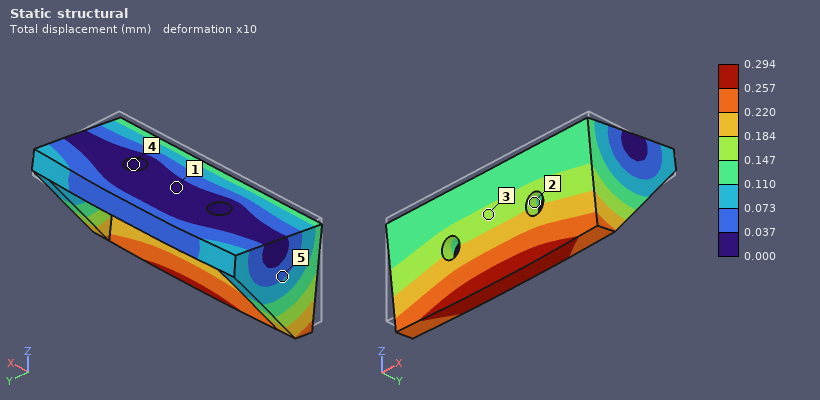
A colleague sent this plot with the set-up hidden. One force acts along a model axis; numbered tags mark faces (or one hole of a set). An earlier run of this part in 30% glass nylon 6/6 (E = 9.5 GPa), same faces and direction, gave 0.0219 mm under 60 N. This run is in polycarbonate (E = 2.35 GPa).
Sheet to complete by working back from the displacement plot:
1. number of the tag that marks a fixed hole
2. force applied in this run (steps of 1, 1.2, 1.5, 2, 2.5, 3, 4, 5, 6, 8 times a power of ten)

4
200 N
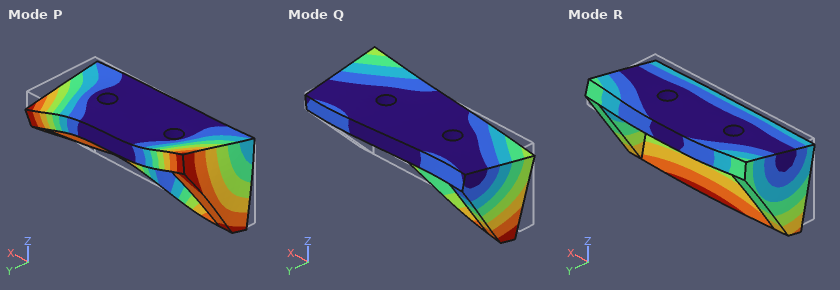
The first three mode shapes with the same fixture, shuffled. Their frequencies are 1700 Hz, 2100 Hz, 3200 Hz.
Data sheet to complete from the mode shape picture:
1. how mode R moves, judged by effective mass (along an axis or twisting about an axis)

along Y
